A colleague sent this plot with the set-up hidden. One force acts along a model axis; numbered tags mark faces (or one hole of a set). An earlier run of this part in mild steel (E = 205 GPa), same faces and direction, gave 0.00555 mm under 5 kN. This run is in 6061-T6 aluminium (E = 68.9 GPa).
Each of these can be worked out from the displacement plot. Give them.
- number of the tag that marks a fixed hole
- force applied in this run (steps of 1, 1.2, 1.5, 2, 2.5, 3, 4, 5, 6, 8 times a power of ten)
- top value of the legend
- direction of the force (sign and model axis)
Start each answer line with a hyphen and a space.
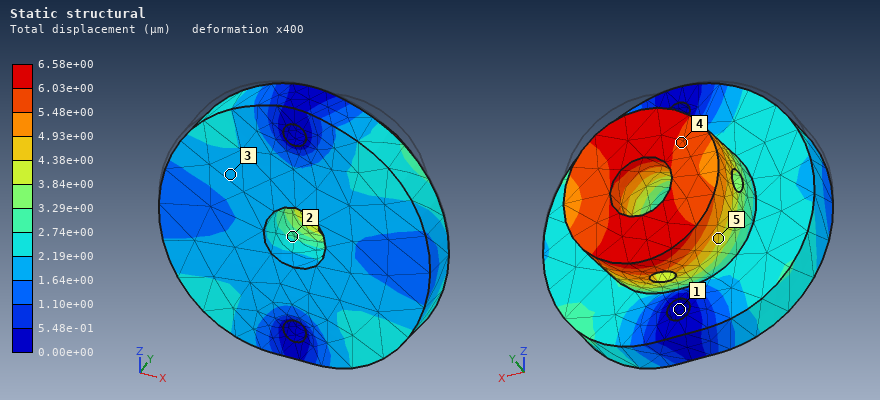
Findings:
- 1
- 2 kN
- 6.58e+00 µm
- -Z
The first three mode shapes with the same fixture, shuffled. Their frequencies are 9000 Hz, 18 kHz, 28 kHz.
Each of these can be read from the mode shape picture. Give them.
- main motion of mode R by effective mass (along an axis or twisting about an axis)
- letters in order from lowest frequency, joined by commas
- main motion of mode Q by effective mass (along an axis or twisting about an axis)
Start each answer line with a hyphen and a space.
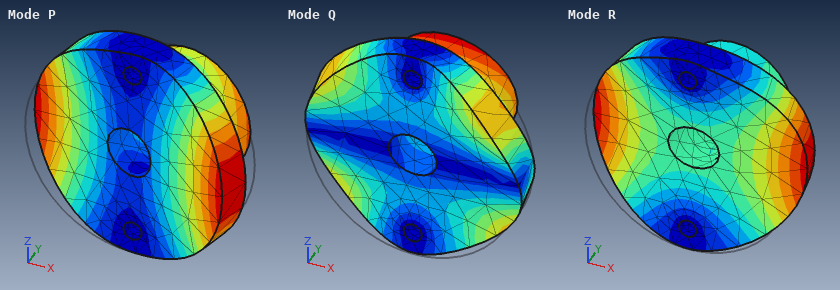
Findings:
- along Y
- P, R, Q
- along Z
